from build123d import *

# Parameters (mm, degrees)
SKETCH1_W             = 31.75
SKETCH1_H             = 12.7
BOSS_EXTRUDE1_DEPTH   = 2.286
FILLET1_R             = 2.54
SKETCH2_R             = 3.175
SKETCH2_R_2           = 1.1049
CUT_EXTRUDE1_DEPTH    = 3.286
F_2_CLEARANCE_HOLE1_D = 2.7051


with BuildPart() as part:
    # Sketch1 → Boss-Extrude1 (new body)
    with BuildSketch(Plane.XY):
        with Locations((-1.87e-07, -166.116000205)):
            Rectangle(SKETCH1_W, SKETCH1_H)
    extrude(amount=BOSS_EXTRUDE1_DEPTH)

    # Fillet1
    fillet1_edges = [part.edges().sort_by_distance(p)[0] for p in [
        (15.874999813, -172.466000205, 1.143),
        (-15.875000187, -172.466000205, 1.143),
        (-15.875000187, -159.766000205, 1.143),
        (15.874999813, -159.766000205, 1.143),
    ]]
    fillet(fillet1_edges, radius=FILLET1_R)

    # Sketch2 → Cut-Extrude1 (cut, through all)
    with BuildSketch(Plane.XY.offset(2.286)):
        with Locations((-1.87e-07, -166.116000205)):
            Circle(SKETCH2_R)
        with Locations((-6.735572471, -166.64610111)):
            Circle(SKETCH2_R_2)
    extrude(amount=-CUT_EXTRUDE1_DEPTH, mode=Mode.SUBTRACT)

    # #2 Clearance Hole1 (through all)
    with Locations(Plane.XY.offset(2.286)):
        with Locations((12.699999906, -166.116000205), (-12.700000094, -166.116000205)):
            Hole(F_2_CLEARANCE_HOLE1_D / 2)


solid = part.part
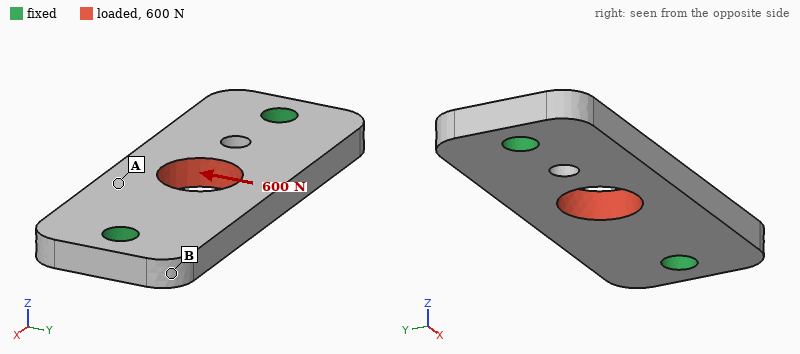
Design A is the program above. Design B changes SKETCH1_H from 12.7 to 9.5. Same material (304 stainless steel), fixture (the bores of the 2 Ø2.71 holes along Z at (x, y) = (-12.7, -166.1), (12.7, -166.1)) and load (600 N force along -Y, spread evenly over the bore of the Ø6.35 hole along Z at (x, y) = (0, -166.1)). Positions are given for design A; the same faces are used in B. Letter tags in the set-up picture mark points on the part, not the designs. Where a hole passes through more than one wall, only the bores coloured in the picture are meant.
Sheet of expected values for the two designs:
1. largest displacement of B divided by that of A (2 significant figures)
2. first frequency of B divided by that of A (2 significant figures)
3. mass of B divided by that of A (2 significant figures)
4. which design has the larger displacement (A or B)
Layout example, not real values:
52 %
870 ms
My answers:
1.6
1.1
0.71
B
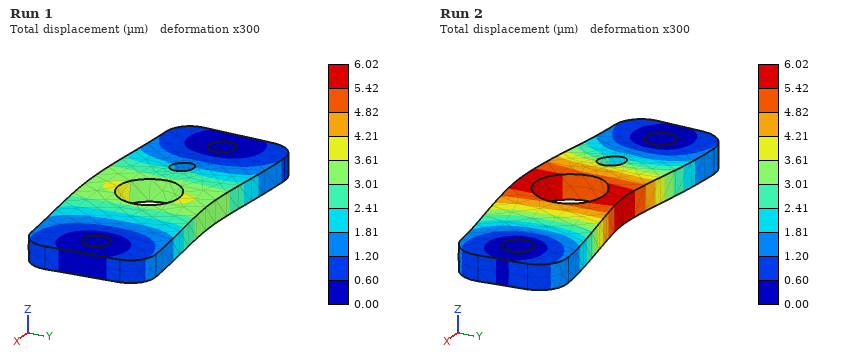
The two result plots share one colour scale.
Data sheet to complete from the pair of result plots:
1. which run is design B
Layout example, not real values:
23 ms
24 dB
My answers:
Run 2
